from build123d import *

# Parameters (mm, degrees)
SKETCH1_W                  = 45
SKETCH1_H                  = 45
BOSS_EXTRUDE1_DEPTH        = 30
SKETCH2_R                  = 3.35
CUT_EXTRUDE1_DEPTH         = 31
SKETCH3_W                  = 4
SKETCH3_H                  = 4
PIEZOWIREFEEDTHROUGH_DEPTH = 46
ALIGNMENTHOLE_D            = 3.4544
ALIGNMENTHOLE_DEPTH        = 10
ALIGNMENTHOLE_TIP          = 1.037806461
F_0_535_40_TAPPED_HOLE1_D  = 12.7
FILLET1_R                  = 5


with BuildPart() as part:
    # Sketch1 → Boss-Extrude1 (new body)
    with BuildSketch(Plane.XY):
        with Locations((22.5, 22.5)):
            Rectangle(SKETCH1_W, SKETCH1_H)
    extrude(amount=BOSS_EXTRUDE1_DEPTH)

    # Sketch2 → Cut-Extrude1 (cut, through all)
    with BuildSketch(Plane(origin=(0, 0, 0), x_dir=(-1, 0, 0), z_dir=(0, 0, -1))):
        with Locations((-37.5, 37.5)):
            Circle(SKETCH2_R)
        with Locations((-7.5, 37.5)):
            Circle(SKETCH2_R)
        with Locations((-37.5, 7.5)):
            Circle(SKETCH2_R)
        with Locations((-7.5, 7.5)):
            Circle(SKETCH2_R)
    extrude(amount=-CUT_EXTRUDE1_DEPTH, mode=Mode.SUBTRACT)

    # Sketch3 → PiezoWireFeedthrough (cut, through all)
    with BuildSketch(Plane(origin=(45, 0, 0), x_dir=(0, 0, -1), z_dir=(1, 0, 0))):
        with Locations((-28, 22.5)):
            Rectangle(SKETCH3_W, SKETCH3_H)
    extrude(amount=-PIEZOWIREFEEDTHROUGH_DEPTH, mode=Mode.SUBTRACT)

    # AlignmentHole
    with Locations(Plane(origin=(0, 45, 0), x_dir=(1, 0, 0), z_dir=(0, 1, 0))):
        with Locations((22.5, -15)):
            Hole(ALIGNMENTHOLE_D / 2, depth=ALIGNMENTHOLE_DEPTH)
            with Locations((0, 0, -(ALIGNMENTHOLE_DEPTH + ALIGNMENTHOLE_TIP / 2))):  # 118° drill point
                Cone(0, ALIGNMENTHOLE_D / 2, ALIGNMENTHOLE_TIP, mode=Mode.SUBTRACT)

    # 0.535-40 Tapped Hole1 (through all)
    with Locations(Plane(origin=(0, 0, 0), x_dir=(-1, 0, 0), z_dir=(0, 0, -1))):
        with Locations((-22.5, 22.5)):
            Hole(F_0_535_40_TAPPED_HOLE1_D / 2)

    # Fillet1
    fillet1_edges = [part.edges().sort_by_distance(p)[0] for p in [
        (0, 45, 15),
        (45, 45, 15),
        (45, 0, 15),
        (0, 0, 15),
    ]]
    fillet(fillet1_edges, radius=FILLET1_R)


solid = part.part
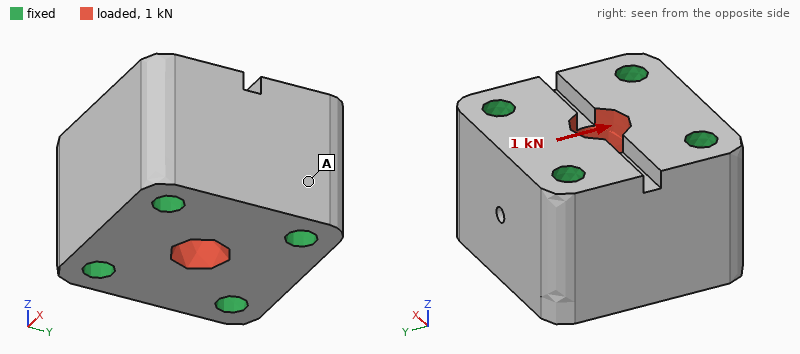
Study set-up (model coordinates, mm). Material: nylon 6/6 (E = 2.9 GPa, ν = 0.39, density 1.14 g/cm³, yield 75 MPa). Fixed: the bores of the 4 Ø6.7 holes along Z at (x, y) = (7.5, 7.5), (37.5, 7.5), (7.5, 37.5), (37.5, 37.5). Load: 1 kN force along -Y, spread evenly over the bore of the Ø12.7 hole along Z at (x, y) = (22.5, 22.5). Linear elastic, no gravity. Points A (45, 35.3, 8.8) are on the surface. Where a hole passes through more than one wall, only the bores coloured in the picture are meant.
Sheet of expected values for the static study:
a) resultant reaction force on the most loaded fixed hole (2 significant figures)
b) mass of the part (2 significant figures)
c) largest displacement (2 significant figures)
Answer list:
280 N
59 g
6.1 µm
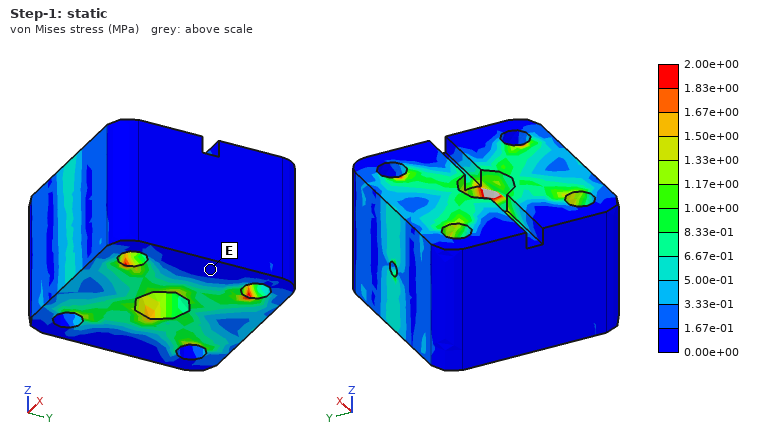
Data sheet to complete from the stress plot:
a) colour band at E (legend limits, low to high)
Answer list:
0.00e+00 to 1.67e-01 MPa
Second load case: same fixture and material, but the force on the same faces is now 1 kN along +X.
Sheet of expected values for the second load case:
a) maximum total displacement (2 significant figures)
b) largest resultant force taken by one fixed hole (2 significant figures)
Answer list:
6.0 µm
280 N
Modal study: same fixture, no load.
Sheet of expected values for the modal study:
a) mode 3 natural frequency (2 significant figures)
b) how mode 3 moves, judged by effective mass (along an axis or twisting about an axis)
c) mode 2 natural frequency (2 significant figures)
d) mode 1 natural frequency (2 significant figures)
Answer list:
16 kHz
along Y
15 kHz
15 kHz
